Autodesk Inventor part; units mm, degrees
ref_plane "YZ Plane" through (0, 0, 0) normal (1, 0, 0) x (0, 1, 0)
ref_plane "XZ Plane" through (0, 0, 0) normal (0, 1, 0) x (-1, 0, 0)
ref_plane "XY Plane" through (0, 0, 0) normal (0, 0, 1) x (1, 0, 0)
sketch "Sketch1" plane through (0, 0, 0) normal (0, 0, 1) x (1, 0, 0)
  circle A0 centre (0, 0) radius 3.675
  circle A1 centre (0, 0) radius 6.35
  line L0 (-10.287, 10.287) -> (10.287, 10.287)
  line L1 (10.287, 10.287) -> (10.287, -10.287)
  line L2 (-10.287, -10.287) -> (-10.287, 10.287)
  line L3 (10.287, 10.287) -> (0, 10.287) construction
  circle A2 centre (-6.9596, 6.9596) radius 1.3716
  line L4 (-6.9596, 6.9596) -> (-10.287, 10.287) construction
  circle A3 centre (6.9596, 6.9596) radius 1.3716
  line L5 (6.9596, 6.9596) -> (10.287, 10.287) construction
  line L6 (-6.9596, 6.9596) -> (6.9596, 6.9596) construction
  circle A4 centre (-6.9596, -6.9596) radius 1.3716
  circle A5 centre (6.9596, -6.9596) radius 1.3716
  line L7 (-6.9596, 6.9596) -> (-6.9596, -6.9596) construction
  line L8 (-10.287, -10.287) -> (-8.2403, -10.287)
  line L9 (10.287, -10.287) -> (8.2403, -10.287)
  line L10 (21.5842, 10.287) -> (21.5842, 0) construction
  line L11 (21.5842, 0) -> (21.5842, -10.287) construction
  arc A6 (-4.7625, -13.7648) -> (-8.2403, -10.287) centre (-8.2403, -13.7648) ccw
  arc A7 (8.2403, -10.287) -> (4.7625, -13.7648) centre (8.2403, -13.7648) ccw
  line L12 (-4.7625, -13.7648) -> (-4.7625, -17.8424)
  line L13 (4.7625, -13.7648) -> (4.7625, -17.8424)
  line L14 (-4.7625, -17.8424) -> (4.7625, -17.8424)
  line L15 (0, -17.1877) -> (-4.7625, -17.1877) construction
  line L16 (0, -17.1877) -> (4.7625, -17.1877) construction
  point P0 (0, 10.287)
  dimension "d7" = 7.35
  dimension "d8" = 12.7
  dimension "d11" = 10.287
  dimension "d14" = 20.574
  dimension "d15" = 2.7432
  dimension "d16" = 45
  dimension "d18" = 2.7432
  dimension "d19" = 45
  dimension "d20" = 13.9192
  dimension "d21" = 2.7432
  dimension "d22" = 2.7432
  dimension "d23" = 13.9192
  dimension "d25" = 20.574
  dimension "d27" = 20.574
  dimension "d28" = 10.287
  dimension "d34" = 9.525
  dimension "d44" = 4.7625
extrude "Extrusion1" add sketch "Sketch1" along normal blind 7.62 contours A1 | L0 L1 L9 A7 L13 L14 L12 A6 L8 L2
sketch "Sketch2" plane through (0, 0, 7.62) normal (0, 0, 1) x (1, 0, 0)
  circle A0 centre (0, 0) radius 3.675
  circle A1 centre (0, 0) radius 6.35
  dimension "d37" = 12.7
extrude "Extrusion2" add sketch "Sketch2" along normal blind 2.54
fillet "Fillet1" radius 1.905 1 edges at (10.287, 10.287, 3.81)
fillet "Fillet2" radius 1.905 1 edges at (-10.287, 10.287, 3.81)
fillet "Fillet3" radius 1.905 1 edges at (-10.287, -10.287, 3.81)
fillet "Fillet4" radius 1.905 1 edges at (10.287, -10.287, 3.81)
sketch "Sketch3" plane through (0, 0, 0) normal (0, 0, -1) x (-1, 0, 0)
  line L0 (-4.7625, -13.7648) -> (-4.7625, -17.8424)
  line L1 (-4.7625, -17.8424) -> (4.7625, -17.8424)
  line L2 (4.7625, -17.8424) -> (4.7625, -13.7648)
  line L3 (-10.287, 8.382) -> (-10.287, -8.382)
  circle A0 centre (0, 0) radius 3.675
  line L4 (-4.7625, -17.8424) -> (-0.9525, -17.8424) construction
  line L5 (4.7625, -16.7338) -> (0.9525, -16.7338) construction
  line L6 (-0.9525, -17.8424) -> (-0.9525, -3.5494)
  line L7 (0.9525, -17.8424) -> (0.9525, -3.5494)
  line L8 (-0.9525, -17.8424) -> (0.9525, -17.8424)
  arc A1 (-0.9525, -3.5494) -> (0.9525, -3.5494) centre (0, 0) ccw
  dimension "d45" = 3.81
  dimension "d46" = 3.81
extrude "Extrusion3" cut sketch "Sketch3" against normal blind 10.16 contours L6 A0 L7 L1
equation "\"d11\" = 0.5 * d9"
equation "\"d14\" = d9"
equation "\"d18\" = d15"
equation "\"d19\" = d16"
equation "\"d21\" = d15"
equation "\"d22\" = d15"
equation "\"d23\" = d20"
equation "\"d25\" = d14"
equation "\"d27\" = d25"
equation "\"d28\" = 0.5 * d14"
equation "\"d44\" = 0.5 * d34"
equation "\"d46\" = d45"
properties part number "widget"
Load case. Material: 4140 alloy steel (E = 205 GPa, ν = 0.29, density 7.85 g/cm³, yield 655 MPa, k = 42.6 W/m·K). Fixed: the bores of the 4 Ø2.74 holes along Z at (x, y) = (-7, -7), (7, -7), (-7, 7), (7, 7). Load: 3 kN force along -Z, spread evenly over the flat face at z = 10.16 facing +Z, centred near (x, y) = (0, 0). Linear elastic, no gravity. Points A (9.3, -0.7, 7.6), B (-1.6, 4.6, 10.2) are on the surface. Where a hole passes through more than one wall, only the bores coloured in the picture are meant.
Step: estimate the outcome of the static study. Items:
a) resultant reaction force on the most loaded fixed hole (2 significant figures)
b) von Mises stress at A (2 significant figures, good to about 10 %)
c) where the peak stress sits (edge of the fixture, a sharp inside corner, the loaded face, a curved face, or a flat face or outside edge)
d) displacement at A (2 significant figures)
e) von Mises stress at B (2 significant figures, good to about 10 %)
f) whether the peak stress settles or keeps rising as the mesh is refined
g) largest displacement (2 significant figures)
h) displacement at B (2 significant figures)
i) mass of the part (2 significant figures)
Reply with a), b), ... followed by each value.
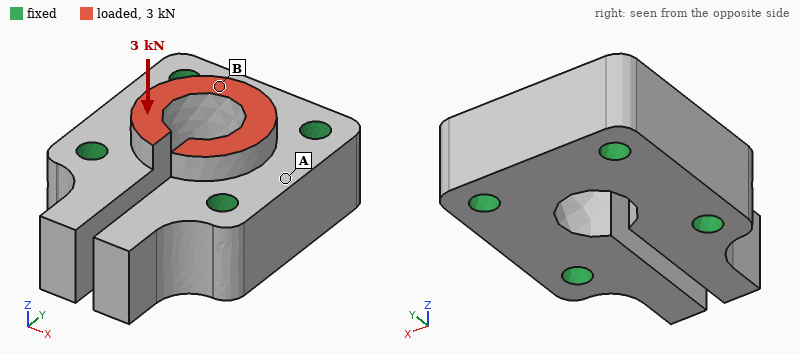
a) 800 N
b) 11 MPa
c) edge of the fixture
d) 0.46 µm
e) 32 MPa
f) keeps rising
g) 2.6 µm
h) 1.6 µm
i) 26 g
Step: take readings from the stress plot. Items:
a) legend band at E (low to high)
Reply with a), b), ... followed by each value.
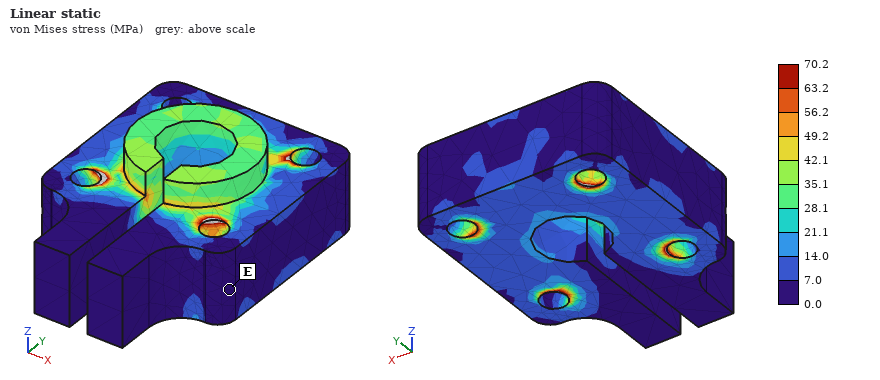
a) 0.0 to 7.0 MPa
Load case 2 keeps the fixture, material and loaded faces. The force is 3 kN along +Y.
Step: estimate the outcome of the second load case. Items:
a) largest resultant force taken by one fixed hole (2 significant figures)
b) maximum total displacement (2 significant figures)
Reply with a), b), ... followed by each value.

a) 980 N
b) 5.6 µm
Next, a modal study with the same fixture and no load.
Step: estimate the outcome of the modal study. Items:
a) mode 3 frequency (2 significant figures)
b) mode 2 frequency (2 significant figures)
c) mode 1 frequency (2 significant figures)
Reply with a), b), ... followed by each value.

a) 43 kHz
b) 37 kHz
c) 37 kHz
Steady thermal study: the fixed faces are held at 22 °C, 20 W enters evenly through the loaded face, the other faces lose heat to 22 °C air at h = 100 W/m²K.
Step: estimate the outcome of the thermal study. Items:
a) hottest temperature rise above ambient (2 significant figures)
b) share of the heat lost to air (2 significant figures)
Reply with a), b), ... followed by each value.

a) 31 K
b) 4.4 %
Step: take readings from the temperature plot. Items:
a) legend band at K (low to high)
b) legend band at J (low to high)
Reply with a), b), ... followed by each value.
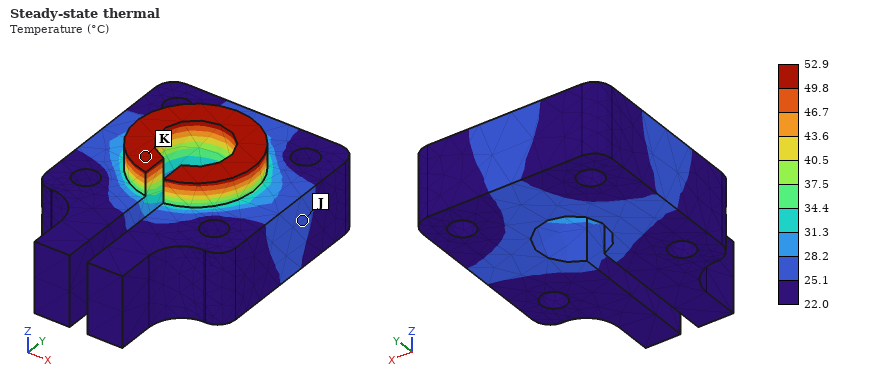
a) 49.8 to 52.9 °C
b) 25.1 to 28.2 °C
